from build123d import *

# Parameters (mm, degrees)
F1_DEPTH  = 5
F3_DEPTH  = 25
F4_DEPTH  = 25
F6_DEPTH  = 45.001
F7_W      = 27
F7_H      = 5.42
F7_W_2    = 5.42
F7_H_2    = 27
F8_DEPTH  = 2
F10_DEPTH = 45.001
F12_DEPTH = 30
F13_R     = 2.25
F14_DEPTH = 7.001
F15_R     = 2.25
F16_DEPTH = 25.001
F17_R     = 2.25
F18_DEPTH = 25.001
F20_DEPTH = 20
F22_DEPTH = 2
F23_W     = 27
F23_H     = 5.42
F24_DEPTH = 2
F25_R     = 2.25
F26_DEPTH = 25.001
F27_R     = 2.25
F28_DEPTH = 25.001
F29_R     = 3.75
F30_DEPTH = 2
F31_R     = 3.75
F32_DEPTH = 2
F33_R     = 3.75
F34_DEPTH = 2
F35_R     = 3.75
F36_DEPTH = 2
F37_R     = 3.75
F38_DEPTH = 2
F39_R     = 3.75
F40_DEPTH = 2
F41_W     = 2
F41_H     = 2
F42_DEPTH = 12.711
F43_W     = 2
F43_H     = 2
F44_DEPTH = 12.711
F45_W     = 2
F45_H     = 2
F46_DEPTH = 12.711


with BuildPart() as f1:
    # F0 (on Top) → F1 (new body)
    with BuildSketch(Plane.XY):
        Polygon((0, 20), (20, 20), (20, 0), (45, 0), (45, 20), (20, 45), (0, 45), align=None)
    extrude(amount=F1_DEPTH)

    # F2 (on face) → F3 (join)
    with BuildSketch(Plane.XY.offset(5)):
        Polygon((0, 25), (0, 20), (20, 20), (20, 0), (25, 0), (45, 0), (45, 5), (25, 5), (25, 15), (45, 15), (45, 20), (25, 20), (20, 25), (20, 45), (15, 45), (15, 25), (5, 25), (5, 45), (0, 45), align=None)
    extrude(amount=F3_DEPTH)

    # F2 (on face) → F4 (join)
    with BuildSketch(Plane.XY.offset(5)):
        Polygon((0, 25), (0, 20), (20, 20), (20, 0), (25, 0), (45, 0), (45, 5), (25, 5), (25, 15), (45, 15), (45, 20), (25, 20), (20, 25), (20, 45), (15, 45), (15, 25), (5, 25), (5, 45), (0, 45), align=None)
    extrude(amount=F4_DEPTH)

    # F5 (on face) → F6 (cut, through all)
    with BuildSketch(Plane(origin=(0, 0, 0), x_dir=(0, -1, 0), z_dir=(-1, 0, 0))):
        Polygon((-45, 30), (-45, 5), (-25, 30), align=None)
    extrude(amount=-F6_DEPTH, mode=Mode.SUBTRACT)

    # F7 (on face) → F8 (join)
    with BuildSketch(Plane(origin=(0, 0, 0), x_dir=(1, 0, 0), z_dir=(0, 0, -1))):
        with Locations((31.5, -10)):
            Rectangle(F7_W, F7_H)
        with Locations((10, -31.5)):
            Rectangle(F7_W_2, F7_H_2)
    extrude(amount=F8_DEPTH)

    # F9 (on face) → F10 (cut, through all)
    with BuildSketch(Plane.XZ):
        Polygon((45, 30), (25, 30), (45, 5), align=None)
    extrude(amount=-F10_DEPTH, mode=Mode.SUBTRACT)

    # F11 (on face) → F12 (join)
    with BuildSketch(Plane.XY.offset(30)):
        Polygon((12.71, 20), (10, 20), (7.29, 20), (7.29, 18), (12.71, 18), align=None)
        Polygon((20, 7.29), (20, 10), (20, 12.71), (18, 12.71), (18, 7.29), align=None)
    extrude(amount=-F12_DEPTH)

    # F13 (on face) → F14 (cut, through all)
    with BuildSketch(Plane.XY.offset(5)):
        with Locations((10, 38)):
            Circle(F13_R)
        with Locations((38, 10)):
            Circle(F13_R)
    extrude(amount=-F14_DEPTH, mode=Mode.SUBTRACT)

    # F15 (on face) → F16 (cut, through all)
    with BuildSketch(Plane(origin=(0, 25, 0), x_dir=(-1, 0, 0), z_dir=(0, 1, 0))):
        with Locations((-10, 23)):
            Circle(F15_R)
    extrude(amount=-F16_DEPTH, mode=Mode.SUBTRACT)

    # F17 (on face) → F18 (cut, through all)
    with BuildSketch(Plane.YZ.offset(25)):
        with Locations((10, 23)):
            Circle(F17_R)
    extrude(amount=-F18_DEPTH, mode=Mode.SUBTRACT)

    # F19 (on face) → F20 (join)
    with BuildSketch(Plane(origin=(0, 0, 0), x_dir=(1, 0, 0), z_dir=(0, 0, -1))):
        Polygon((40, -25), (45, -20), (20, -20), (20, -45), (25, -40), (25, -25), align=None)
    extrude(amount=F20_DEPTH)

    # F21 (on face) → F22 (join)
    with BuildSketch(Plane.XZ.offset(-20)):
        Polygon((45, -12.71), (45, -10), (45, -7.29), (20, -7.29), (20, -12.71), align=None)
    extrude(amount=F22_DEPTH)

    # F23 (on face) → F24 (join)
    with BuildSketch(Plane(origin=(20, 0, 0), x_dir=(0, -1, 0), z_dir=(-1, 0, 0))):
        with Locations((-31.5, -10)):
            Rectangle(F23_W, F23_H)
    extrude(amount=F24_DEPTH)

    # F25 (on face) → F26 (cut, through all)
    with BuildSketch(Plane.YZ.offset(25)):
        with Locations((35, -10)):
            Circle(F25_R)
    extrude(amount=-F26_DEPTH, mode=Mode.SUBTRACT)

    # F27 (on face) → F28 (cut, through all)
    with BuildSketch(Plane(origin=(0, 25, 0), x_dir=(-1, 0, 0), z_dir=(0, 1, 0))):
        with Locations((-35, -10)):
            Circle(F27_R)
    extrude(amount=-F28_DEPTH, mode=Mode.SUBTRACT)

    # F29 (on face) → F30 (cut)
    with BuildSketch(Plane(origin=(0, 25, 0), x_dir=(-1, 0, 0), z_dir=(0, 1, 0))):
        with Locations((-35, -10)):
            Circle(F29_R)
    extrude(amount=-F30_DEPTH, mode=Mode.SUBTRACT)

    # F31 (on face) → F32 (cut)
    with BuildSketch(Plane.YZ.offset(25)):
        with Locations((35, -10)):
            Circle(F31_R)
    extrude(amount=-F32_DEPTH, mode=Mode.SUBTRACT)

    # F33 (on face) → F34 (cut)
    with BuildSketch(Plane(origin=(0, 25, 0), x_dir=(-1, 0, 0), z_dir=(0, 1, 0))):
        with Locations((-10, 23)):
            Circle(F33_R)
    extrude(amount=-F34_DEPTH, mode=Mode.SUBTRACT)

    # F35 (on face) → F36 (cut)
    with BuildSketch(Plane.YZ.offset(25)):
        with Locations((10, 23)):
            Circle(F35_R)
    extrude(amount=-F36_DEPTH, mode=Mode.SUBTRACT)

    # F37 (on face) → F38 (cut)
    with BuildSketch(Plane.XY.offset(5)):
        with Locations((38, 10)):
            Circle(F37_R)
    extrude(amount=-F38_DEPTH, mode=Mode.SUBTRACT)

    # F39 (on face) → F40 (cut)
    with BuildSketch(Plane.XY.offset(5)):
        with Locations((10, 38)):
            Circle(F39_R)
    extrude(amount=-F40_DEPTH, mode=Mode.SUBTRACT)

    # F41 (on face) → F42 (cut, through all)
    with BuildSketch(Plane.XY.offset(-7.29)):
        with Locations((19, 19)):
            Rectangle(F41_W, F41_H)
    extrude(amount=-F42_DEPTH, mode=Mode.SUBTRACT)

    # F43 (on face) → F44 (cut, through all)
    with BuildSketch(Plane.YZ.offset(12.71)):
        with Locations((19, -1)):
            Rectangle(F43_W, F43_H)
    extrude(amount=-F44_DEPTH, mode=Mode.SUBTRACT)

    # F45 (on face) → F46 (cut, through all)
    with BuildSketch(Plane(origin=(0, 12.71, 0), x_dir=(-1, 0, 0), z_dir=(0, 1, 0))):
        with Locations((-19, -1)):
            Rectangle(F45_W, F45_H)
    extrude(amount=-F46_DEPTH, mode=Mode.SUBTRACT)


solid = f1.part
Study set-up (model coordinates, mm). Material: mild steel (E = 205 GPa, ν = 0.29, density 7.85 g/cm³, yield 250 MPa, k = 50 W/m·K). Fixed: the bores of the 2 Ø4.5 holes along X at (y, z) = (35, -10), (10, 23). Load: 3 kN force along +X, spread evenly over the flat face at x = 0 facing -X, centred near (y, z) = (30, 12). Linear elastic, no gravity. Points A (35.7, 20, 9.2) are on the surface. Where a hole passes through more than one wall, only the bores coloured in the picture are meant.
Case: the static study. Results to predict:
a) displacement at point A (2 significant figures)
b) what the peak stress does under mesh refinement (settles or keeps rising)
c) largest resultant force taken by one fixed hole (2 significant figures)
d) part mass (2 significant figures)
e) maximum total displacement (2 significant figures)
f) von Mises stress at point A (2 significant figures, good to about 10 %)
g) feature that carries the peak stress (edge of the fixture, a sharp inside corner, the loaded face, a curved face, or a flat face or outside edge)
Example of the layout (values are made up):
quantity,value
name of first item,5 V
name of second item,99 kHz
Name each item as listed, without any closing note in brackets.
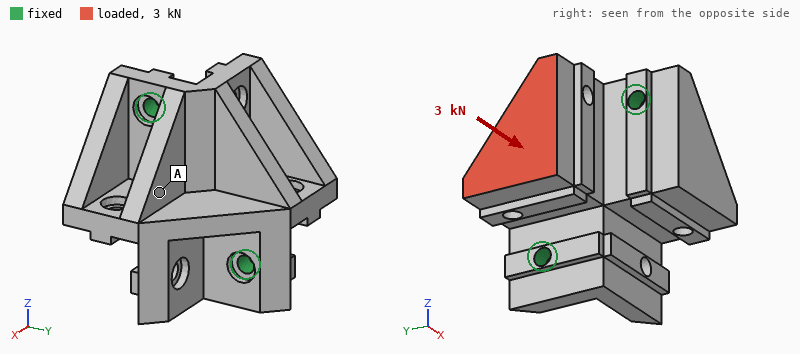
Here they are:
quantity,value
displacement at point A,18 µm
what the peak stress does under mesh refinement,keeps rising
largest resultant force taken by one fixed hole,1.6 kN
part mass,170 g
maximum total displacement,57 µm
von Mises stress at point A,26 MPa
feature that carries the peak stress,edge of the fixture
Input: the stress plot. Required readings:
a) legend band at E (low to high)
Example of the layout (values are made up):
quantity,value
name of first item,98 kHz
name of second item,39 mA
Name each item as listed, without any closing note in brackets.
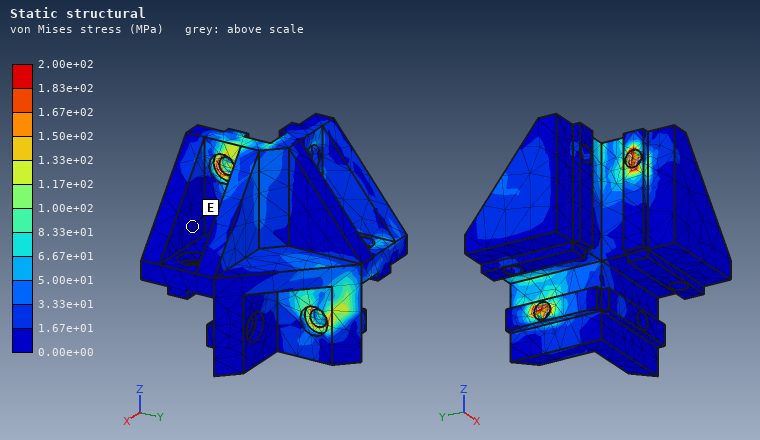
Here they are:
quantity,value
legend band at E,0.00e+00 to 1.67e+01 MPa
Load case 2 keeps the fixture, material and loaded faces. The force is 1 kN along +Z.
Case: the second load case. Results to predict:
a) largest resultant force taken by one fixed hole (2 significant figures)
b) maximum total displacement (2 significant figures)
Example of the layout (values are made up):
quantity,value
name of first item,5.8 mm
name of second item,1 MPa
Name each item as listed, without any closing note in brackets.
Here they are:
quantity,value
largest resultant force taken by one fixed hole,700 N
maximum total displacement,26 µm
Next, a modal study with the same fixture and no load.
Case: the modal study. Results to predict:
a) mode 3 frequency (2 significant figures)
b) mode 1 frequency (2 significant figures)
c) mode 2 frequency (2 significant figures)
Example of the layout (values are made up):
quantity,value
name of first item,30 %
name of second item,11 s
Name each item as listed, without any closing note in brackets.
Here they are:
quantity,value
mode 3 frequency,9300 Hz
mode 1 frequency,3700 Hz
mode 2 frequency,7500 Hz
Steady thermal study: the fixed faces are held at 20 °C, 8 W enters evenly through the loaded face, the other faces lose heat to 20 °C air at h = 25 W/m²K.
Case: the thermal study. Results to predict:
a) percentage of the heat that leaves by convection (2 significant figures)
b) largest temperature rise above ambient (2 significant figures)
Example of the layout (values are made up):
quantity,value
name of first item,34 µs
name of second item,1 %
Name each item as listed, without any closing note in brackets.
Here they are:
quantity,value
percentage of the heat that leaves by convection,22 %
largest temperature rise above ambient,22 K
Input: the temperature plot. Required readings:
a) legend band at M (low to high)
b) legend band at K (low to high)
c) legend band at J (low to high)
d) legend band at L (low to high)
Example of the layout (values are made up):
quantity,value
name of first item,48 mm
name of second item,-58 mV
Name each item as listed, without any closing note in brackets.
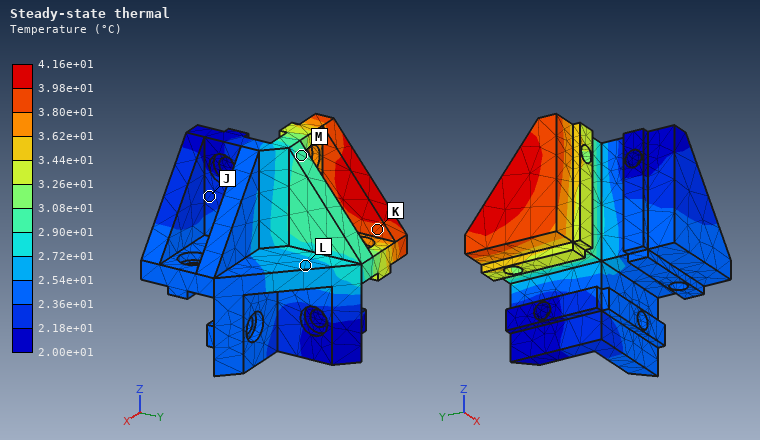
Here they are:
quantity,value
legend band at M,2.90e+01 to 3.08e+01 °C
legend band at K,3.80e+01 to 3.98e+01 °C
legend band at J,2.18e+01 to 2.36e+01 °C
legend band at L,2.54e+01 to 2.72e+01 °C
